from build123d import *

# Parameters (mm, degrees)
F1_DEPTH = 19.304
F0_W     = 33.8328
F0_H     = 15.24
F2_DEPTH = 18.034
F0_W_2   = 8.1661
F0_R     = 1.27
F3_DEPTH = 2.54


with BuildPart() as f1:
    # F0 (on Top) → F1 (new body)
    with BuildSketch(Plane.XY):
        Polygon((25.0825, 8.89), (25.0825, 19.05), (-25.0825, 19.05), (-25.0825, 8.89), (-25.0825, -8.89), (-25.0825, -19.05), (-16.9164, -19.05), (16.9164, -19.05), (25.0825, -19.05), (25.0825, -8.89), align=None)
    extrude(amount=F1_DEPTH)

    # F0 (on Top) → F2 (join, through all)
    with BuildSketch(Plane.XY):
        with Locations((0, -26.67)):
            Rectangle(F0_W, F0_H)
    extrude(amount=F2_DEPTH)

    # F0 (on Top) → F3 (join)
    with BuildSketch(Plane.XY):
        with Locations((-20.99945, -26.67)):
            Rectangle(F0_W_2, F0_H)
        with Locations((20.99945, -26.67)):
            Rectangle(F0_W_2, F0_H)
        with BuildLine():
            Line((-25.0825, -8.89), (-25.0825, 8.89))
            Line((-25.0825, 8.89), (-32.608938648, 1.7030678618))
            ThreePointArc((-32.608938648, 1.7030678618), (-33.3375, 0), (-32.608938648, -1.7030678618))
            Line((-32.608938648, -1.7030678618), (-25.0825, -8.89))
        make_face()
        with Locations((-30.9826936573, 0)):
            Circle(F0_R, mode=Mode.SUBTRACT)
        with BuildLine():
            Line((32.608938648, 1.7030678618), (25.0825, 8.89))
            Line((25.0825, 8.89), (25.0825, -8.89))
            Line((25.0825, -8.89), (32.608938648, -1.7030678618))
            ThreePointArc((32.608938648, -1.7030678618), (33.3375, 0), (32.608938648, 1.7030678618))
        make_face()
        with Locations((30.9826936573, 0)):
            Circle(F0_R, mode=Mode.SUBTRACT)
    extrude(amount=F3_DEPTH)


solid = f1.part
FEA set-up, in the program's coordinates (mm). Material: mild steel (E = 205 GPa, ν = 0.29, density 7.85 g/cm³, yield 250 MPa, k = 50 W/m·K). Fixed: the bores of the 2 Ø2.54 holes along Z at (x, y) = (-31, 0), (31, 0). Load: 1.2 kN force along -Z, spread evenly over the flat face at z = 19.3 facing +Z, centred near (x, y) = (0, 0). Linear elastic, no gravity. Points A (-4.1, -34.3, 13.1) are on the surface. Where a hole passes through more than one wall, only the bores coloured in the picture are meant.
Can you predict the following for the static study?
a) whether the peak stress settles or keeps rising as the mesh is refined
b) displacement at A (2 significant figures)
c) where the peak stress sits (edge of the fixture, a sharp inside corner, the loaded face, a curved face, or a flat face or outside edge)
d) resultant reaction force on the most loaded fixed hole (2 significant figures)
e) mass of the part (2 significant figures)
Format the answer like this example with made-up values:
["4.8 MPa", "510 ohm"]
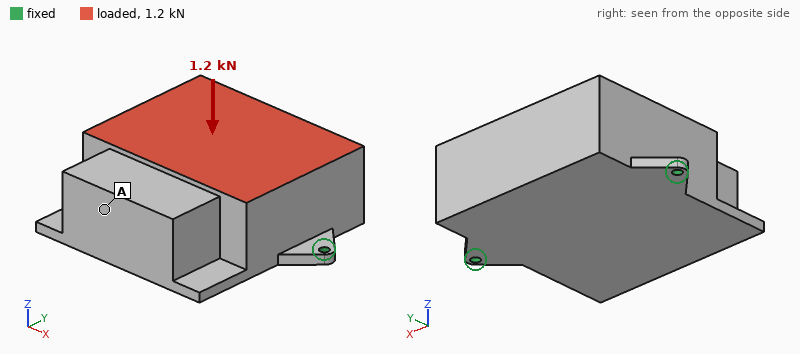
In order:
["keeps rising", "8.7 µm", "edge of the fixture", "670 N", "370 g"]
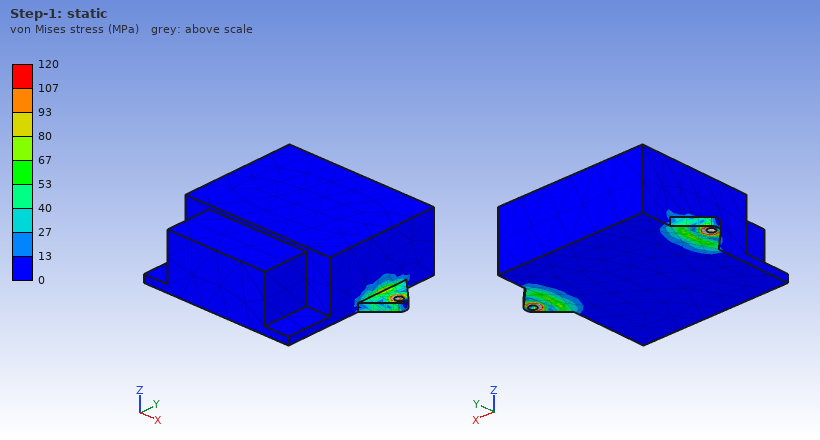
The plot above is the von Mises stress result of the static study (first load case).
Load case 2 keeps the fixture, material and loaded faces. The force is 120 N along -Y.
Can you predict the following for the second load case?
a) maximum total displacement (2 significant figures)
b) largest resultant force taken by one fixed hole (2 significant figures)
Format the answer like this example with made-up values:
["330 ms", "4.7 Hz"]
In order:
["49 µm", "60 N"]
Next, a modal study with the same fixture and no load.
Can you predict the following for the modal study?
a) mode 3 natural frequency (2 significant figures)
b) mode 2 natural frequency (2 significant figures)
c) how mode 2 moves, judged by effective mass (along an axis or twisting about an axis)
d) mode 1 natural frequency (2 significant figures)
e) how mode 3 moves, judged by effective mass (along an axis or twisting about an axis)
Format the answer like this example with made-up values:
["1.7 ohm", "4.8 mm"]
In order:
["5100 Hz", "3300 Hz", "along Z", "580 Hz", "along X"]
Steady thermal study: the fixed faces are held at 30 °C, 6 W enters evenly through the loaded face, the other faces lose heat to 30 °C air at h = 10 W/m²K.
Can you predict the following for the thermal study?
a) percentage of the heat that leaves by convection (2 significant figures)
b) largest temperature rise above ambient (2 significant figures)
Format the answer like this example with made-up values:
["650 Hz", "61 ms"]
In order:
["19 %", "16 K"]
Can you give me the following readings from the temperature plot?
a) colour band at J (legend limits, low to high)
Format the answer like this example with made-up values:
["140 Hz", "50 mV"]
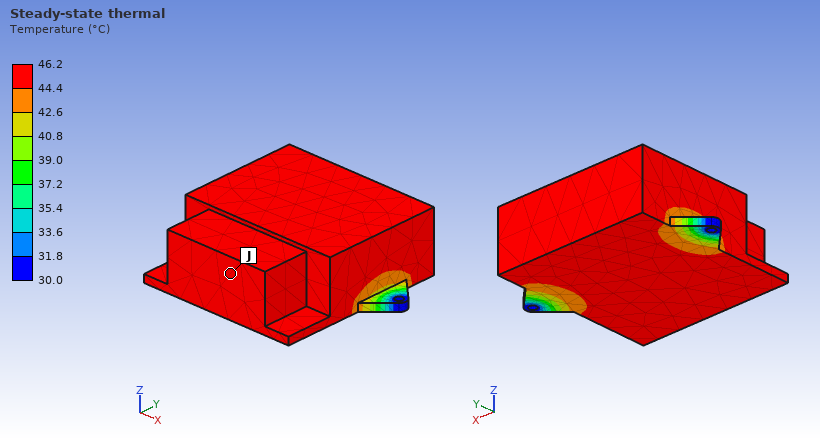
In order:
["44.4 to 46.2 °C"]
